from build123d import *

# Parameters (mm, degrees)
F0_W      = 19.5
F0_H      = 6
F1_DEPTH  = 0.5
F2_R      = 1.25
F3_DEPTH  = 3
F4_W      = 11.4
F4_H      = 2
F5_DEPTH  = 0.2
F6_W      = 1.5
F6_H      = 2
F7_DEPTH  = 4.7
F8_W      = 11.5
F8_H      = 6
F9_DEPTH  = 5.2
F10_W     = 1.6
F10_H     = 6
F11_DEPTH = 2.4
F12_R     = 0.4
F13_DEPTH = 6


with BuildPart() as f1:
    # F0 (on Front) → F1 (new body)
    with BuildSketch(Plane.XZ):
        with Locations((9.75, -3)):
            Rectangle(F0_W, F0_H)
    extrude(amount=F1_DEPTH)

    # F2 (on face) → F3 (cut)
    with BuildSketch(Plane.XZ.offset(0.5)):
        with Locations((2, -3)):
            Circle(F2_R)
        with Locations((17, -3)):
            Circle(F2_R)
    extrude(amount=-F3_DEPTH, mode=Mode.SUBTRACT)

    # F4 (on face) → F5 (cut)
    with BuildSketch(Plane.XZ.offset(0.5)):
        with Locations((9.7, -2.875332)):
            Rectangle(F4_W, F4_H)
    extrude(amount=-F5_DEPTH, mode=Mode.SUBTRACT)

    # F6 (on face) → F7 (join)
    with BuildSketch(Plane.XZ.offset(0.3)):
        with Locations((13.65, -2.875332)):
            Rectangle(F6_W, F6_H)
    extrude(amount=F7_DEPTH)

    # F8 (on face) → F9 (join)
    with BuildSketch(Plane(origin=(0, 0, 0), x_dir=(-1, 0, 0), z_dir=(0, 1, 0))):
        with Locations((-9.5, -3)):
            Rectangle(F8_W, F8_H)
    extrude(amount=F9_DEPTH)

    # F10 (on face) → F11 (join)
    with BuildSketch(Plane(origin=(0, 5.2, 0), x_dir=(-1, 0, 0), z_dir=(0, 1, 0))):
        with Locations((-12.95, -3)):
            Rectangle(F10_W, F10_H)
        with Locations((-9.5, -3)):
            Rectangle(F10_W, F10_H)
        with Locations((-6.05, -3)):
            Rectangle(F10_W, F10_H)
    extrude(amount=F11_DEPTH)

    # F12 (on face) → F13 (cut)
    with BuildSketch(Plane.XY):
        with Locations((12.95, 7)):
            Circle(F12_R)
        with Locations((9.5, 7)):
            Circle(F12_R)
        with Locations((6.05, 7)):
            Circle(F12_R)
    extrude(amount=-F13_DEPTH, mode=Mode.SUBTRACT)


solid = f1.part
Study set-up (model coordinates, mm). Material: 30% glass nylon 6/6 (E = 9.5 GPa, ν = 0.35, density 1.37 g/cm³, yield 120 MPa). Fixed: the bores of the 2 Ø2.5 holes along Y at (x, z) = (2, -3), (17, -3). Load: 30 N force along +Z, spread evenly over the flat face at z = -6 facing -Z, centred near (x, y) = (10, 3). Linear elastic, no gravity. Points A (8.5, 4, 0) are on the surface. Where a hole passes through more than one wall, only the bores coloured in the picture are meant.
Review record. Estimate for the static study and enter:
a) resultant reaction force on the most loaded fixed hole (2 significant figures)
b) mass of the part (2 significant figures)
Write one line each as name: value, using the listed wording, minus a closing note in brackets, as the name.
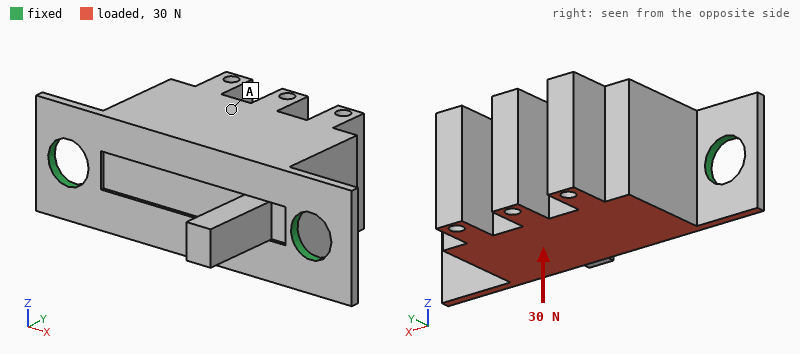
resultant reaction force on the most loaded fixed hole: 15 N
mass of the part: 0.66 g
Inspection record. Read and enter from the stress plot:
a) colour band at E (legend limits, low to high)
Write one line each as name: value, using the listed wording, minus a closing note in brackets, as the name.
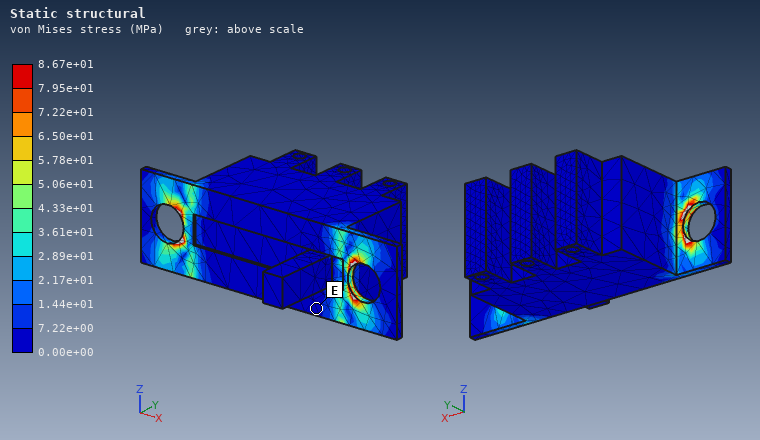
colour band at E: 0.00e+00 to 7.22e+00 MPa
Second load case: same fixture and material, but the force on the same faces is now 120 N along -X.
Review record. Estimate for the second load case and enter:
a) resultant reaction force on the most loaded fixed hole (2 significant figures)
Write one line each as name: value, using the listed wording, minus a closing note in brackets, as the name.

resultant reaction force on the most loaded fixed hole: 71 N
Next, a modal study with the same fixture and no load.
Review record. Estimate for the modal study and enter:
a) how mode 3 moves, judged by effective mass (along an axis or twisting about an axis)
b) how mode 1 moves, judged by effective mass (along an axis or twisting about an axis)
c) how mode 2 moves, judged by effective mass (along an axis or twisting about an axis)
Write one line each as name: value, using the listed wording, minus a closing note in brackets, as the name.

how mode 3 moves, judged by effective mass: along X
how mode 1 moves, judged by effective mass: along Z
how mode 2 moves, judged by effective mass: along Y
